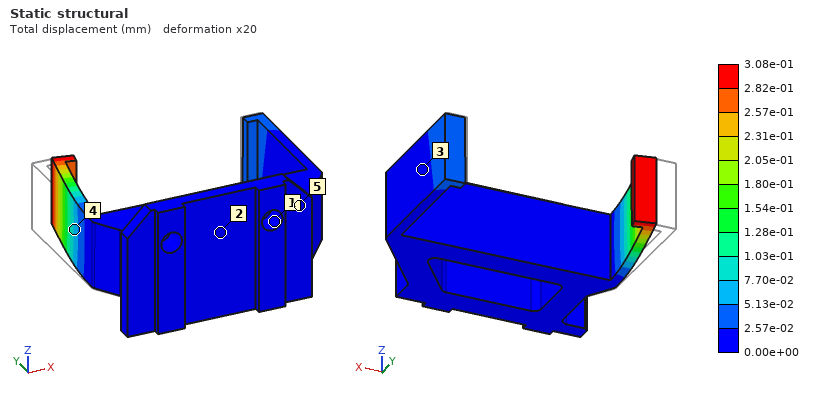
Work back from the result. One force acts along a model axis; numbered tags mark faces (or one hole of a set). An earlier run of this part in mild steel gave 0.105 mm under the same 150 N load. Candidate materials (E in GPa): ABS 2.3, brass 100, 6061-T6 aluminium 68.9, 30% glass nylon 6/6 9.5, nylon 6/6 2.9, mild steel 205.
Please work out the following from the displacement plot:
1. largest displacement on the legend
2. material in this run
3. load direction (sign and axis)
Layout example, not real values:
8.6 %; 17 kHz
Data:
3.08e-01 mm; 6061-T6 aluminium; +X
